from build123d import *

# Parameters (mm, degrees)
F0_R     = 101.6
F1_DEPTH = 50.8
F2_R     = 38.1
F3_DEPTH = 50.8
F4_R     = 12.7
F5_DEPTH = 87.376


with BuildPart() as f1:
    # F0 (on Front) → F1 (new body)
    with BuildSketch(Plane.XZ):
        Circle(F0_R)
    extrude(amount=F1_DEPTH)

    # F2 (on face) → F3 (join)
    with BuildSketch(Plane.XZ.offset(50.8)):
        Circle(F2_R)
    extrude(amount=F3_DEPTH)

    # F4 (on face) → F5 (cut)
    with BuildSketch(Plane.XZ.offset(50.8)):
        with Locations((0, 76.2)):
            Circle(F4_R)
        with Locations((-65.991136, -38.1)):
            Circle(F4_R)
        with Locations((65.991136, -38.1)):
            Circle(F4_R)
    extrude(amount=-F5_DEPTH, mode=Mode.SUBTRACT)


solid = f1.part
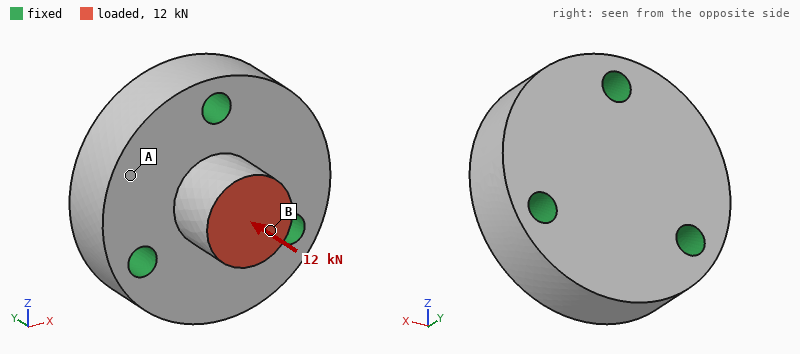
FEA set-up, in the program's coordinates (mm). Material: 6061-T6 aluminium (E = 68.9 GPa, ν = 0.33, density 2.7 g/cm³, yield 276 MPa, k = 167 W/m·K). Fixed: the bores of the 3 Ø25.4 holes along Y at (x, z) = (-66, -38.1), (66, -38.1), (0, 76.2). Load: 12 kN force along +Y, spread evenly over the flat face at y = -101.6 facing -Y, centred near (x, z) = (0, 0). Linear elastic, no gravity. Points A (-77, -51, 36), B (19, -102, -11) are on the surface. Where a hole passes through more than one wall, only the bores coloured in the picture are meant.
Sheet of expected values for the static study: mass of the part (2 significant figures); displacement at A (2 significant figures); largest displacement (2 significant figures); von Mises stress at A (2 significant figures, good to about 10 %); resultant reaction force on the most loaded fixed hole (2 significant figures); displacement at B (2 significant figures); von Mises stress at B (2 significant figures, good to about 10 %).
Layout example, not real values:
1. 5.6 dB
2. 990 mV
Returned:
1. 4.9 kg
2. 1.00 µm
3. 4.7 µm
4. 0.68 MPa
5. 4.1 kN
6. 4.6 µm
7. 2.7 MPa
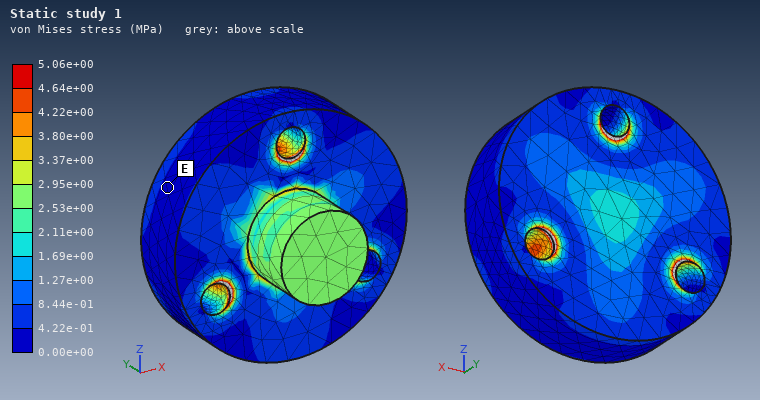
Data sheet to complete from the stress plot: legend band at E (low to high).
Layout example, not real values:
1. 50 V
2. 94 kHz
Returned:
1. 0.00e+00 to 4.22e-01 MPa
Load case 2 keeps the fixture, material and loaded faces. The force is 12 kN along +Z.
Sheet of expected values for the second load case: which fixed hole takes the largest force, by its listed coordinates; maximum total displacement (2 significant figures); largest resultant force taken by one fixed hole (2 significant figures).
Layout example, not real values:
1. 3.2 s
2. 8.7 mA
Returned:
1. (0, 76.2)
2. 23 µm
3. 8.8 kN
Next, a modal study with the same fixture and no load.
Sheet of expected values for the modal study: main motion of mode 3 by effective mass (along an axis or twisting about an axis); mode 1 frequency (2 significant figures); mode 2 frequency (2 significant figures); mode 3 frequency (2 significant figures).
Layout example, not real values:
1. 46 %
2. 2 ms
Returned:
1. along Y
2. 6300 Hz
3. 6300 Hz
4. 7000 Hz
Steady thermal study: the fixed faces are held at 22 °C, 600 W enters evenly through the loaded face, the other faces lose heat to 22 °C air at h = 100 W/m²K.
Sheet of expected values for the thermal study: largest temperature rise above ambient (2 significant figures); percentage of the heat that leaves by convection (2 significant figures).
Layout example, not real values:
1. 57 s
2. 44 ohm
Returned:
1. 58 K
2. 14 %
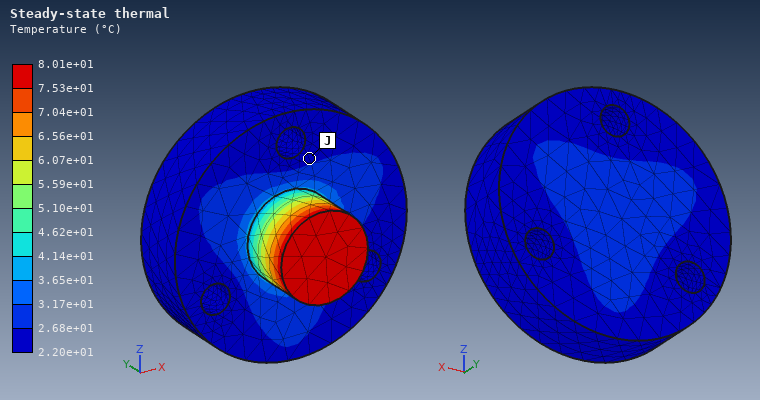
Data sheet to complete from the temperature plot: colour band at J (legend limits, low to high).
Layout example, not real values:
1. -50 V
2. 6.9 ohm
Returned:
1. 2.20e+01 to 2.68e+01 °C
